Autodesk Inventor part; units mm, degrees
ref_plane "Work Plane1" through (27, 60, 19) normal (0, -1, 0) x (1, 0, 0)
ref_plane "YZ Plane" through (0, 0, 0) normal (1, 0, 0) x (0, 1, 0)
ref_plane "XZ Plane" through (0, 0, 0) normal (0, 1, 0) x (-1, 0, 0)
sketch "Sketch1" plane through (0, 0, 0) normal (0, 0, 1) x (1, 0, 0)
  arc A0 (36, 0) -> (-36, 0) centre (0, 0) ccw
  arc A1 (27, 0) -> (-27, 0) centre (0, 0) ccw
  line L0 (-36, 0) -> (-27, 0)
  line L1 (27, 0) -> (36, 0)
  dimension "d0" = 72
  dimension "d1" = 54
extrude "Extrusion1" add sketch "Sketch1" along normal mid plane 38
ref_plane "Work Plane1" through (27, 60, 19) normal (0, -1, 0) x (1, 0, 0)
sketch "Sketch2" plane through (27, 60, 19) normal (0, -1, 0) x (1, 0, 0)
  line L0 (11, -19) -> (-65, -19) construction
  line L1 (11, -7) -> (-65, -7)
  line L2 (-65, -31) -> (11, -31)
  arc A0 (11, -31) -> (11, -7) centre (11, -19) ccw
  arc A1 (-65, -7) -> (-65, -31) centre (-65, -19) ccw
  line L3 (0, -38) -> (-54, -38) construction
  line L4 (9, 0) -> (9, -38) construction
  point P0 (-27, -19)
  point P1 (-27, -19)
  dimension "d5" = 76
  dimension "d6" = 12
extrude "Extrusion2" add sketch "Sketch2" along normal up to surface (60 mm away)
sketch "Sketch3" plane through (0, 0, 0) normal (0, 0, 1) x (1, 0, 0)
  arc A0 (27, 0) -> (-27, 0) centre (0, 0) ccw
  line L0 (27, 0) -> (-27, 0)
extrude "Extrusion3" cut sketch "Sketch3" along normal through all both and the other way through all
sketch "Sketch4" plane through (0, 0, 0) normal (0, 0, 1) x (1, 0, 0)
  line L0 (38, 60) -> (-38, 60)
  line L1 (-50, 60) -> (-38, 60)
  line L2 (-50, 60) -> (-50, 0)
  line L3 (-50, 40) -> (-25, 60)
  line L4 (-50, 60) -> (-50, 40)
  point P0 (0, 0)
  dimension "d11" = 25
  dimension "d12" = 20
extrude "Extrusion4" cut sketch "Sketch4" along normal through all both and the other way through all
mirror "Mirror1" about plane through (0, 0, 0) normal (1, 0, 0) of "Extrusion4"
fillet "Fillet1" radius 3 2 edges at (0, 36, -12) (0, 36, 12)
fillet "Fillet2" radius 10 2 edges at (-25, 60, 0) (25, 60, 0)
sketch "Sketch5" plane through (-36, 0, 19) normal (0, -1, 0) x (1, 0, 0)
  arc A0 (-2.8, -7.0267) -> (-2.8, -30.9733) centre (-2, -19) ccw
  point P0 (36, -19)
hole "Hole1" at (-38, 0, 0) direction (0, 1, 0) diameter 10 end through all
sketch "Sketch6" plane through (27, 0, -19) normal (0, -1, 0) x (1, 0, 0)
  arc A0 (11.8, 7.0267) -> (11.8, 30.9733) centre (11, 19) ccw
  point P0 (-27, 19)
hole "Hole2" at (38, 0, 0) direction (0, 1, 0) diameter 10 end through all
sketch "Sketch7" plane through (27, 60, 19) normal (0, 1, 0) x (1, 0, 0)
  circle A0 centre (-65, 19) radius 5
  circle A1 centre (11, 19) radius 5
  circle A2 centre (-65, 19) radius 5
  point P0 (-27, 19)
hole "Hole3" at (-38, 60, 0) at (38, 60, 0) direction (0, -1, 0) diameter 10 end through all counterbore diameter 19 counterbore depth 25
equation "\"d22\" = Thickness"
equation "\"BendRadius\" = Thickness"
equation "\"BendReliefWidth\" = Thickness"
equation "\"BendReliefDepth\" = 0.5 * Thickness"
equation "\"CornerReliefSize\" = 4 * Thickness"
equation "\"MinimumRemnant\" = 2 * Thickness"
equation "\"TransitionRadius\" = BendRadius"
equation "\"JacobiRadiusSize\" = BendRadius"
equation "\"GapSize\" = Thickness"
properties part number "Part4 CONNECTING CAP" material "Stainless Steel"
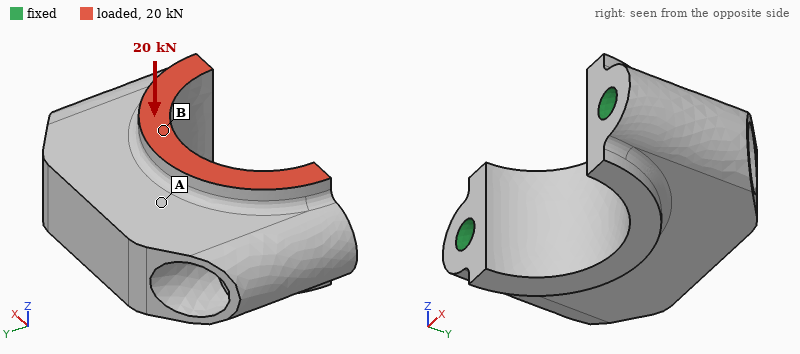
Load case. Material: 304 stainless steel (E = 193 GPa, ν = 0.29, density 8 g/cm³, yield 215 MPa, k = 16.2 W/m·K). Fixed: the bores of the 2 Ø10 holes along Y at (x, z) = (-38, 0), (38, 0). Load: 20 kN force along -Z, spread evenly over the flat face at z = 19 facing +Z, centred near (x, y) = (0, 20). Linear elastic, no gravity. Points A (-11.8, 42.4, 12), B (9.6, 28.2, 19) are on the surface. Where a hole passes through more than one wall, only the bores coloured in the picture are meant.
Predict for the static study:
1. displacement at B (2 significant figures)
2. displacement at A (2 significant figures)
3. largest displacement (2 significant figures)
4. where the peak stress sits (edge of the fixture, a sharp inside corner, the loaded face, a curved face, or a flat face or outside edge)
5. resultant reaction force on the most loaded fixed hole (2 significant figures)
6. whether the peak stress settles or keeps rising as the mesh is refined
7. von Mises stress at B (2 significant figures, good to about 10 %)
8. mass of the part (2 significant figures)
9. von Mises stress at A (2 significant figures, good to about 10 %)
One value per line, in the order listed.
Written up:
6.8 µm
5.7 µm
7.3 µm
edge of the fixture
10 kN
keeps rising
26 MPa
790 g
11 MPa
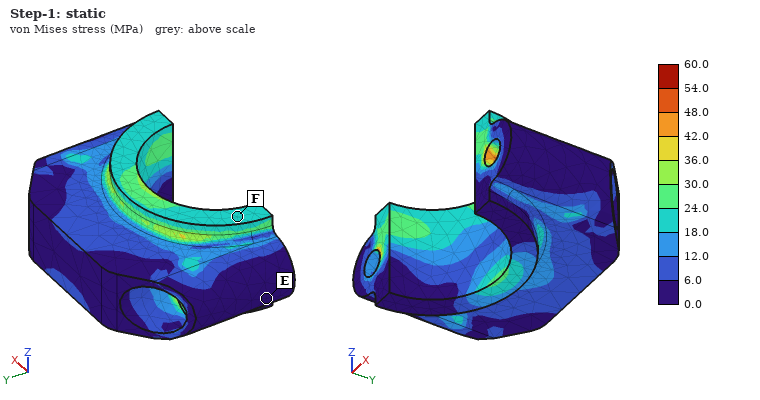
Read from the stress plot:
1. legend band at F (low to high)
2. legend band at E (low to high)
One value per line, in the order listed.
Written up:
18.0 to 24.0 MPa
0.0 to 6.0 MPa
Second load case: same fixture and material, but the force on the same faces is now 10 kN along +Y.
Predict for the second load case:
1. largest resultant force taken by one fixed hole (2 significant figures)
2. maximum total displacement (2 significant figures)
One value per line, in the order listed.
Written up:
5.3 kN
9.1 µm
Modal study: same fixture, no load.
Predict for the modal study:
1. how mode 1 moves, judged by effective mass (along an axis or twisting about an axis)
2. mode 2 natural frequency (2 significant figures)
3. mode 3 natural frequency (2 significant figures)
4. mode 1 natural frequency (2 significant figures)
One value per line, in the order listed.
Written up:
along Z
16 kHz
16 kHz
7700 Hz
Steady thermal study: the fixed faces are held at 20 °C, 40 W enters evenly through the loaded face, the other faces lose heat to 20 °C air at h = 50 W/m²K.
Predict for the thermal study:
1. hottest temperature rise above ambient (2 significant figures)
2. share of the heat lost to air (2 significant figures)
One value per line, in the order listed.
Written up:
49 K
22 %
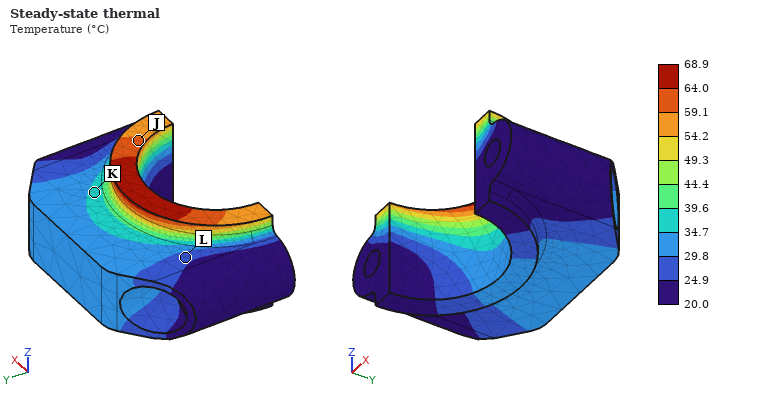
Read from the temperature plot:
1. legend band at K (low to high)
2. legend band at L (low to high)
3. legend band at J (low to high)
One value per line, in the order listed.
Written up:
34.7 to 39.6 °C
24.9 to 29.8 °C
59.1 to 64.0 °C
